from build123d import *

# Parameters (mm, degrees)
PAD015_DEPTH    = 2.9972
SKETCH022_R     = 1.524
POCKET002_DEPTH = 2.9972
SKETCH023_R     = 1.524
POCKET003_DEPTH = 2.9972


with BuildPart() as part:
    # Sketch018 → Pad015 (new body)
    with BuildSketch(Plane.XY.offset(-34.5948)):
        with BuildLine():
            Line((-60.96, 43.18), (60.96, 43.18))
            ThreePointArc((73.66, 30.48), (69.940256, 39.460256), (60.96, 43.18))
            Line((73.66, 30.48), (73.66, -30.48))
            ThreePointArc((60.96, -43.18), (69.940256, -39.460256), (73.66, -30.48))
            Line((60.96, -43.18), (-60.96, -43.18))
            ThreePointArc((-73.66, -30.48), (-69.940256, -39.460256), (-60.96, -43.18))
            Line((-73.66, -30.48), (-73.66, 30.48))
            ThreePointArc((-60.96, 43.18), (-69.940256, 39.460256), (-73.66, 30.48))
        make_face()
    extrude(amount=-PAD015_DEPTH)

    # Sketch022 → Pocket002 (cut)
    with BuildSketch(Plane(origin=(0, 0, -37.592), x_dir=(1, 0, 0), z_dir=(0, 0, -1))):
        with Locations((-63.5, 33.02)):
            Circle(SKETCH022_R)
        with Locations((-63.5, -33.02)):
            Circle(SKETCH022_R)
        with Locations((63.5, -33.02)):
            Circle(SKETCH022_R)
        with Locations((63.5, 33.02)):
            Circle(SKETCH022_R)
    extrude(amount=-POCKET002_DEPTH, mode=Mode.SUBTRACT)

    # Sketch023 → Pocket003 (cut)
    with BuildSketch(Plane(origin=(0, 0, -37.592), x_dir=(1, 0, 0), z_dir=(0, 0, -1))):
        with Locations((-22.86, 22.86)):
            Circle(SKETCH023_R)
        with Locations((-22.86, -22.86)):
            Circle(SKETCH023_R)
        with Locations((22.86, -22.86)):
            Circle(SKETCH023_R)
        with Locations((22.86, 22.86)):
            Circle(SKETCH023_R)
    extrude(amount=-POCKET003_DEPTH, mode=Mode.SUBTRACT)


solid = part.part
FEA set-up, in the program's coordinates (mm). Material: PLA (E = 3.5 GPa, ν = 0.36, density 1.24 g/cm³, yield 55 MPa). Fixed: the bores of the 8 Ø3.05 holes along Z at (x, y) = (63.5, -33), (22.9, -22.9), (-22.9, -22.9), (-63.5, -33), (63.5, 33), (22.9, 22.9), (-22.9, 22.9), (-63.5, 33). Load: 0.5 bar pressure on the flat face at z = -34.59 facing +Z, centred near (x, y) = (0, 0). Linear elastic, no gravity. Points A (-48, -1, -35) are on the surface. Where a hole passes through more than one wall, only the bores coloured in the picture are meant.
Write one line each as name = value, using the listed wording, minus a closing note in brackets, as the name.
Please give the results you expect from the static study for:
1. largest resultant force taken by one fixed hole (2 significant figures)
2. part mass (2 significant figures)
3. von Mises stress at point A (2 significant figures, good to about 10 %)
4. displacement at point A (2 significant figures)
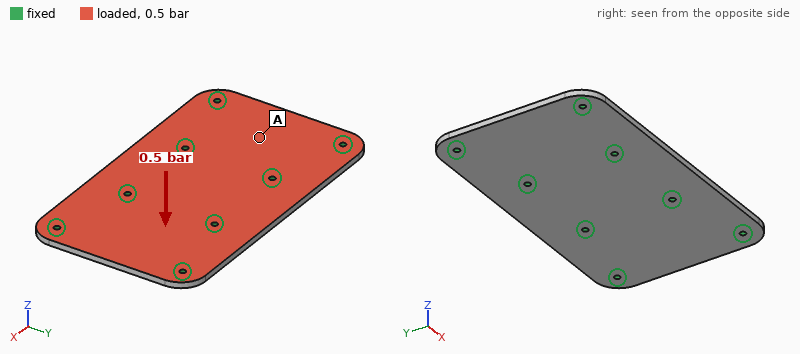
largest resultant force taken by one fixed hole = 98 N
part mass = 47 g
von Mises stress at point A = 4.0 MPa
displacement at point A = 0.25 mm
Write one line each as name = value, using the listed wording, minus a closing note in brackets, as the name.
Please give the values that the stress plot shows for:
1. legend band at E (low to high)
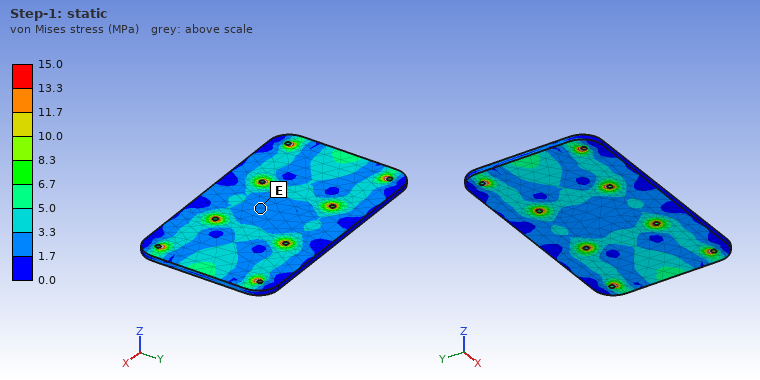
legend band at E = 1.7 to 3.3 MPa
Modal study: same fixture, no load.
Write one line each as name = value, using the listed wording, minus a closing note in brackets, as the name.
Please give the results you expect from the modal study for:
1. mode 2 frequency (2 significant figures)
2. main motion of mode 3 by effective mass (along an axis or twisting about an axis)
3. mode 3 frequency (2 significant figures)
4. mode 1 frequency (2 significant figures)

mode 2 frequency = 1200 Hz
main motion of mode 3 by effective mass = along Z
mode 3 frequency = 1500 Hz
mode 1 frequency = 1200 Hz
